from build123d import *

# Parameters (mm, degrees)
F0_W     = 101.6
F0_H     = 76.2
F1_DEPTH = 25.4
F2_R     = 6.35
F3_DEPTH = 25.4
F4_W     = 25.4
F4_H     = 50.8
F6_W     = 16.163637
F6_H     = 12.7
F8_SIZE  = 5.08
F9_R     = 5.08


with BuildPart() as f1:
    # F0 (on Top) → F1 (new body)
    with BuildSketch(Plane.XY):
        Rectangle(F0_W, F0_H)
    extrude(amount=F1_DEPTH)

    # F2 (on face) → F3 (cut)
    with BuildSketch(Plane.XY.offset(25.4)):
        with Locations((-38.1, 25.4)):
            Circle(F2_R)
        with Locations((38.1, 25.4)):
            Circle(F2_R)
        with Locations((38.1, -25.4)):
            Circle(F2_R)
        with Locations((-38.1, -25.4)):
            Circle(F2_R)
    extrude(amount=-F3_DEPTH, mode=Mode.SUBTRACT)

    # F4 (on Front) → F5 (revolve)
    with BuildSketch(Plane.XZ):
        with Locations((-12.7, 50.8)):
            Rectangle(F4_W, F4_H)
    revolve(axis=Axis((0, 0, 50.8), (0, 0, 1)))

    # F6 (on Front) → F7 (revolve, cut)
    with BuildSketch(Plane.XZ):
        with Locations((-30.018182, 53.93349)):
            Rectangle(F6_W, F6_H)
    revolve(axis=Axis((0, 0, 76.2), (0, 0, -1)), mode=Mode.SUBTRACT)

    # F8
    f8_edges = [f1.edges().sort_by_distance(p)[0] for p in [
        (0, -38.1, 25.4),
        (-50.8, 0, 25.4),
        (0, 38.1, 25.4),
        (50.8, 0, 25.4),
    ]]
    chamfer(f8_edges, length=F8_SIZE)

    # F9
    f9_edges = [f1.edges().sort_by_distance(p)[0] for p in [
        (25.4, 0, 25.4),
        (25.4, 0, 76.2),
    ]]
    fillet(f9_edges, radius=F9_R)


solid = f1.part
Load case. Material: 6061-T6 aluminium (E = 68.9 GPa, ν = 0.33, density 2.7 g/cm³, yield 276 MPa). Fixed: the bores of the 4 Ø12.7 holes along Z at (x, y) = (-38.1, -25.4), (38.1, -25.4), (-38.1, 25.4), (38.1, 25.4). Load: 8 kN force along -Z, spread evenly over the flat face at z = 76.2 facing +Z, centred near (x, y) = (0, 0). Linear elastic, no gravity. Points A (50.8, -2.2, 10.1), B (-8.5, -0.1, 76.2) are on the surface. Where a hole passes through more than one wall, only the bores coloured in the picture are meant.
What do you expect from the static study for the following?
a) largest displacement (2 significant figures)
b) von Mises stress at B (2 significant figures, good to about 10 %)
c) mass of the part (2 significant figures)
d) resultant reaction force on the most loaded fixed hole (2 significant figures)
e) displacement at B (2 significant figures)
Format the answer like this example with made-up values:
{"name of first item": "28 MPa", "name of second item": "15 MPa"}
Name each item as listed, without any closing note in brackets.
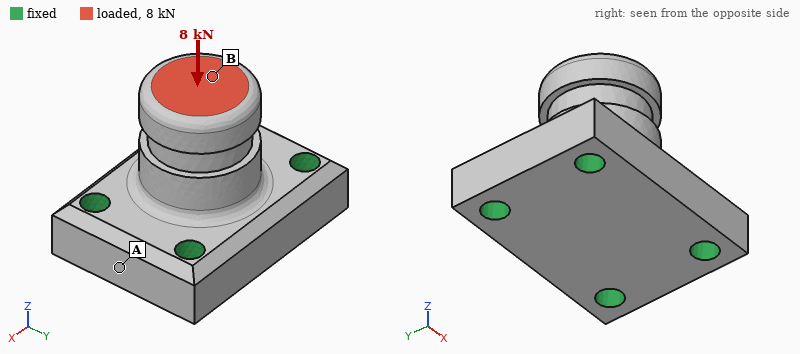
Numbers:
{"largest displacement": "6.8 µm", "von Mises stress at B": "4.4 MPa", "mass of the part": "740 g", "resultant reaction force on the most loaded fixed hole": "2.1 kN", "displacement at B": "6.7 µm"}
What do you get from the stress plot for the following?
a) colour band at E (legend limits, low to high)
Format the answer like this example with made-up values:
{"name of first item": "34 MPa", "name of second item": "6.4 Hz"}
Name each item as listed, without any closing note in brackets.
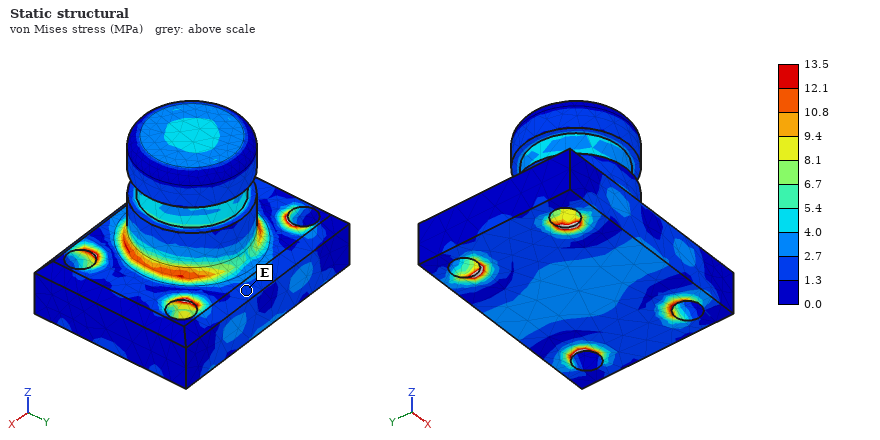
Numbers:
{"colour band at E": "1.3 to 2.7 MPa"}
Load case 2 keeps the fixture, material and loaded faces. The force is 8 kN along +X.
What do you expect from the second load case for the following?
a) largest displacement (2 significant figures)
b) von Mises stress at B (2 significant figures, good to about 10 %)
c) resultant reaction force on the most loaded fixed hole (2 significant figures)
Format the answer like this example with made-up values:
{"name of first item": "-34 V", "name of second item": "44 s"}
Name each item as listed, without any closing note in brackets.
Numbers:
{"largest displacement": "45 µm", "von Mises stress at B": "11 MPa", "resultant reaction force on the most loaded fixed hole": "4.4 kN"}
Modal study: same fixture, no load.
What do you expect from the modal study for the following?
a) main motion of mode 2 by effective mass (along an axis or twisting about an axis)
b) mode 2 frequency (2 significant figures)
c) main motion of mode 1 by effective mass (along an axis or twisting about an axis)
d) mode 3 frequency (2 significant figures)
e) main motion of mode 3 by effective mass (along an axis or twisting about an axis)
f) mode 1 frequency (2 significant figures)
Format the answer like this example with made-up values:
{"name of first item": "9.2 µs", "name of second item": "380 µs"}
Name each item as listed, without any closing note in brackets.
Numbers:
{"main motion of mode 2 by effective mass": "along X", "mode 2 frequency": "7500 Hz", "main motion of mode 1 by effective mass": "along Y", "mode 3 frequency": "11 kHz", "main motion of mode 3 by effective mass": "along Z", "mode 1 frequency": "6400 Hz"}
